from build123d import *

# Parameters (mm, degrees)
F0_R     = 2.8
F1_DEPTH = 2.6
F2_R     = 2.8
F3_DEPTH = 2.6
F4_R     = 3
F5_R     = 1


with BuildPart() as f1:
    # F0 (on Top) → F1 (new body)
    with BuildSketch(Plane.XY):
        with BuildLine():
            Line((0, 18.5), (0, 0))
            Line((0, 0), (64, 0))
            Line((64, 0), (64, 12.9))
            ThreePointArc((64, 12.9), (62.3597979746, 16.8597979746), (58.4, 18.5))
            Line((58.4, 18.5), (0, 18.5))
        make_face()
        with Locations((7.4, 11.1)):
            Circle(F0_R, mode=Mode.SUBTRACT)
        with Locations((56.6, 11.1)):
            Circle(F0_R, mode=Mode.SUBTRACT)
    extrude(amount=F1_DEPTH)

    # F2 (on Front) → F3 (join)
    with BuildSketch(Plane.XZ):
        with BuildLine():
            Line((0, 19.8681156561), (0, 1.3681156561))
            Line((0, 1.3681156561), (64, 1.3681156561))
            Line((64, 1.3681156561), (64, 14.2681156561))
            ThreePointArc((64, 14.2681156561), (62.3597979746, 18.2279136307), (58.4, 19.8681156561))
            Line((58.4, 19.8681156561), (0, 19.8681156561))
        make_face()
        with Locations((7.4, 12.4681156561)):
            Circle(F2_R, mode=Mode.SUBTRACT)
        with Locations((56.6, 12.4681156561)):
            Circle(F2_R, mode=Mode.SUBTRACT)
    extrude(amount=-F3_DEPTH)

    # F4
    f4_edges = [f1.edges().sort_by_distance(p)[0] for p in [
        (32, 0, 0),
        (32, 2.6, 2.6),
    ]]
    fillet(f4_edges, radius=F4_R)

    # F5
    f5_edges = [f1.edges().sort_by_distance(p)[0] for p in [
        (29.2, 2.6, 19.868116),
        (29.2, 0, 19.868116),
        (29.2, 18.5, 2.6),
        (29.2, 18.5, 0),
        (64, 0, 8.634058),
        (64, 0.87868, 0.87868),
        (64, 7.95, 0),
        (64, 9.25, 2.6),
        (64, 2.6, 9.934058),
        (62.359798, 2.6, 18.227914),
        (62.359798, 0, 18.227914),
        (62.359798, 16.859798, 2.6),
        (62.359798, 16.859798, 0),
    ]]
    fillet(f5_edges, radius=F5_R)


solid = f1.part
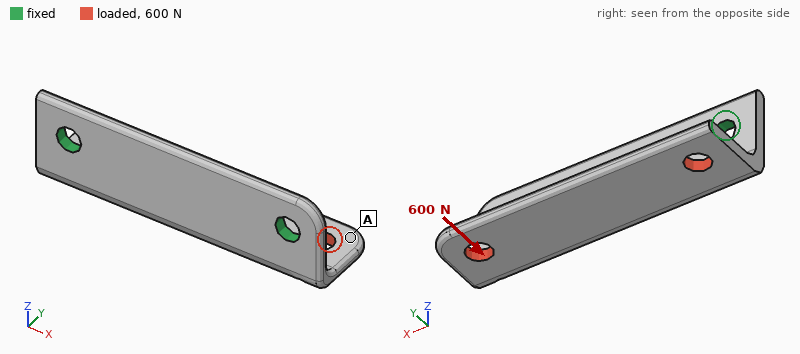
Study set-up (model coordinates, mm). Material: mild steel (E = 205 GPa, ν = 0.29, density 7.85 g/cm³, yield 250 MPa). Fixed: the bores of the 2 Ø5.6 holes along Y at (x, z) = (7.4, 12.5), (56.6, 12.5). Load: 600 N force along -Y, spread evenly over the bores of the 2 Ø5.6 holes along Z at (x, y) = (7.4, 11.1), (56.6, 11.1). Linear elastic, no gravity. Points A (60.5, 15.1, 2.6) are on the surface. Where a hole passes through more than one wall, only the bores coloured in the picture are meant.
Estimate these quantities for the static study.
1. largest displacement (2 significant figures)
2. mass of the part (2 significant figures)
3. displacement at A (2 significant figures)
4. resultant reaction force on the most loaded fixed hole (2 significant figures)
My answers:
40 µm
44 g
32 µm
300 N
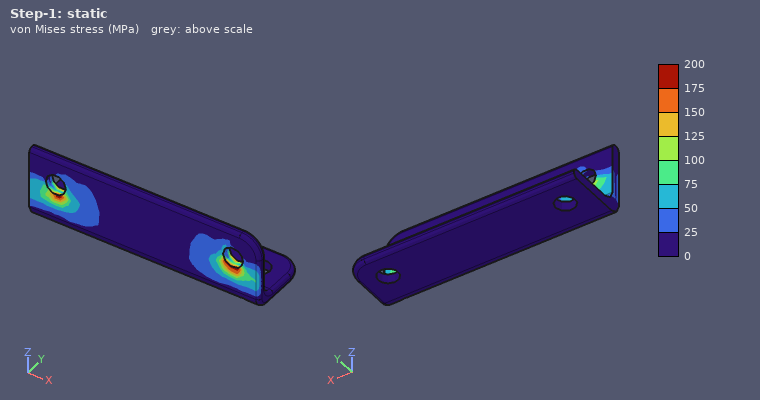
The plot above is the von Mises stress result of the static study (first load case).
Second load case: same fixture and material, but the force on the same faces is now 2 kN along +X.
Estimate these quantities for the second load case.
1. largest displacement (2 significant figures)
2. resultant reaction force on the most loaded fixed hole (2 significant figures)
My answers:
36 µm
1.1 kN
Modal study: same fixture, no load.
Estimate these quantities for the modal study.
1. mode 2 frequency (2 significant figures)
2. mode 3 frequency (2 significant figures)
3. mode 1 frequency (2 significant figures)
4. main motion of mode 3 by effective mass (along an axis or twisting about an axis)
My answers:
6000 Hz
8000 Hz
3700 Hz
along Y
